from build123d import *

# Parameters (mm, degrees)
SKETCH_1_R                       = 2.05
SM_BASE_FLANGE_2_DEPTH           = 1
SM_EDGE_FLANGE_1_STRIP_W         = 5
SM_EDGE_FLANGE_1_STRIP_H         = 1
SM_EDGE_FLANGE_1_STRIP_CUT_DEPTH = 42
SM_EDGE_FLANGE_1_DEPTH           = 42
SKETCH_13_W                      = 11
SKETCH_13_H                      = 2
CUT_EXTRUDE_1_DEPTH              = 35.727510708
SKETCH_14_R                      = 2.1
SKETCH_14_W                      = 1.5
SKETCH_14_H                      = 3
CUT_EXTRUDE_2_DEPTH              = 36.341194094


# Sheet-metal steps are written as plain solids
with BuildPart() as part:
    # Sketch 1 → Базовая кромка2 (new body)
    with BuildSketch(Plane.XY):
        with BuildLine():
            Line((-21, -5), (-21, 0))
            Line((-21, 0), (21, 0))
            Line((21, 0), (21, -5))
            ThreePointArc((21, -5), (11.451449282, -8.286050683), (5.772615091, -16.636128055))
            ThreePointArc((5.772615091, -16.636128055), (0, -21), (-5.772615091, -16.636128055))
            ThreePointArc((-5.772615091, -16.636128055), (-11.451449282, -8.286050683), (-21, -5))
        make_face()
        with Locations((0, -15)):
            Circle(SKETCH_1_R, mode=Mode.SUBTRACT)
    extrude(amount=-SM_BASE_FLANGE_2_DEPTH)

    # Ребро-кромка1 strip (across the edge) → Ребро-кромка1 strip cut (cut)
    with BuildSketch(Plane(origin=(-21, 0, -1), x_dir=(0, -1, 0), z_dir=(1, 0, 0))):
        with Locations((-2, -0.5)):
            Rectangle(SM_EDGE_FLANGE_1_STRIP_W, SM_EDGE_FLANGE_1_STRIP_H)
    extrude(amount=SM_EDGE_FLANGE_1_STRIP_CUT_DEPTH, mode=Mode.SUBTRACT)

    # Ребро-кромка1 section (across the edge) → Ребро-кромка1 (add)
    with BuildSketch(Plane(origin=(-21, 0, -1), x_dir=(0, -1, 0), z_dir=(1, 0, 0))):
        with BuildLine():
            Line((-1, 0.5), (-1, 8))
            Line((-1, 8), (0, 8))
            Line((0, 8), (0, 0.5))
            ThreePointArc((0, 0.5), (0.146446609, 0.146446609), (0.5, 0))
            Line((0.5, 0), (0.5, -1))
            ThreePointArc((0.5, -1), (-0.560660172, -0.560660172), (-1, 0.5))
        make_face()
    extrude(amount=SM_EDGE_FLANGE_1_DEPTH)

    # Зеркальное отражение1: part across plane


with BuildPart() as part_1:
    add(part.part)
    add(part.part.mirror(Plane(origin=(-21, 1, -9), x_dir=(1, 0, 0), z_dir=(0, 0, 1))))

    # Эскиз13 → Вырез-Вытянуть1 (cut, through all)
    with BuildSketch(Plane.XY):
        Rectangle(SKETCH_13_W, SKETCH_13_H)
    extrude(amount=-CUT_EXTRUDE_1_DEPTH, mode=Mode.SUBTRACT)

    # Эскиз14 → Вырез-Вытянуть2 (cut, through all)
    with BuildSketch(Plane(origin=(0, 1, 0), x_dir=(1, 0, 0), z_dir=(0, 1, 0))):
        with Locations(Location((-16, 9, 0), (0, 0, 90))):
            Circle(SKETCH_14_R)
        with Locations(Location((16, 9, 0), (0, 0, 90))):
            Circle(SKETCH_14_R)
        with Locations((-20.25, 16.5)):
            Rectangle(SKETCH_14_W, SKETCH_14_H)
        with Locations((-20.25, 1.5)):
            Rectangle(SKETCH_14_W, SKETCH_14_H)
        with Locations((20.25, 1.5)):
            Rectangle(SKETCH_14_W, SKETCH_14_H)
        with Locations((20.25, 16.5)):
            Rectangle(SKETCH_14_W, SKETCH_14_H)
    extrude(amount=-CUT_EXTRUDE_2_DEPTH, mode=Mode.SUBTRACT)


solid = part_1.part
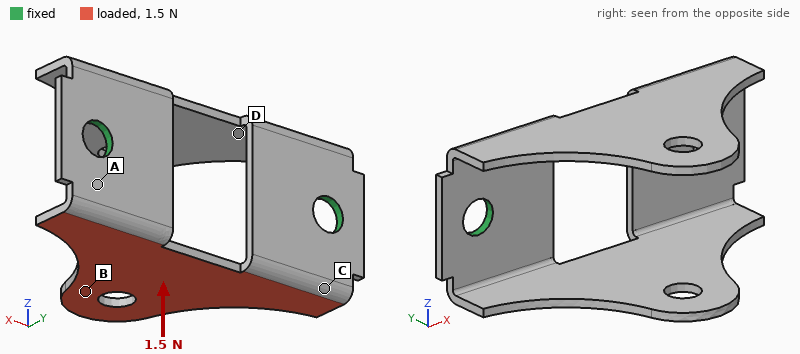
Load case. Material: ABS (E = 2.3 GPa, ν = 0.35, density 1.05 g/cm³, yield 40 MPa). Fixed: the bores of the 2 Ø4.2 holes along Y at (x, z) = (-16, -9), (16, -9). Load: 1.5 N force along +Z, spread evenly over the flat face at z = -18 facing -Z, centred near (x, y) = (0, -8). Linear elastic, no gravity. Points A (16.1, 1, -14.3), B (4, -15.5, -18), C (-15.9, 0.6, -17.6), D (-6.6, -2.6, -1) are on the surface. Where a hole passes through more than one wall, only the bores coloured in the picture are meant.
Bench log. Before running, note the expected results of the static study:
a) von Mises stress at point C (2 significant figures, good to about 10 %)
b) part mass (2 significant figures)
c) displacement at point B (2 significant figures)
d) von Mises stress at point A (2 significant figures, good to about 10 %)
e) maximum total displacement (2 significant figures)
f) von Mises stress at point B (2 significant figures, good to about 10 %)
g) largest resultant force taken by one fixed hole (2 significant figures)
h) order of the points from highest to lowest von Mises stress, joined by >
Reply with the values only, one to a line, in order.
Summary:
1.2 MPa
1.4 g
0.43 mm
2.1 MPa
0.61 mm
0.58 MPa
0.75 N
A > C > B > D
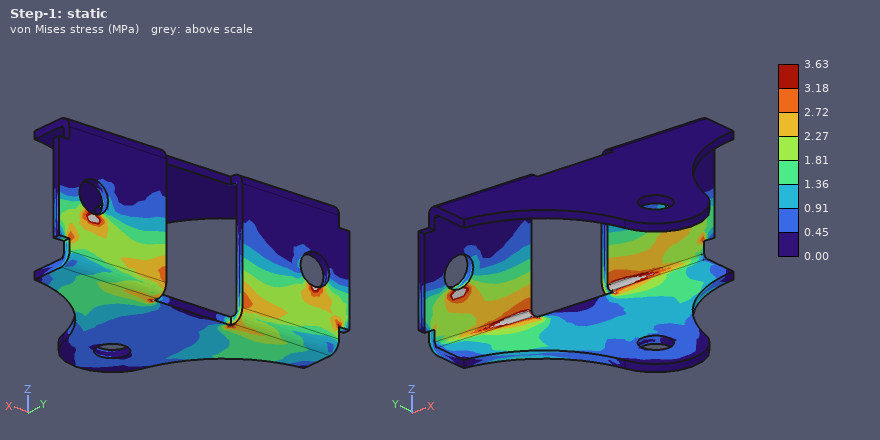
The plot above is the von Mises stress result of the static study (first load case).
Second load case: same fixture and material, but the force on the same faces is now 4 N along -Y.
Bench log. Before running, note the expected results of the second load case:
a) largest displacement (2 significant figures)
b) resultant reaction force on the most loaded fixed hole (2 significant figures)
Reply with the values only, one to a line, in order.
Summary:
0.49 mm
2.3 N
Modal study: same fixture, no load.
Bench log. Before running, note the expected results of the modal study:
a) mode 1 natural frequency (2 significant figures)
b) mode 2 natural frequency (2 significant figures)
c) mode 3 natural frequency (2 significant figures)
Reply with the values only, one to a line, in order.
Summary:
510 Hz
510 Hz
1600 Hz
